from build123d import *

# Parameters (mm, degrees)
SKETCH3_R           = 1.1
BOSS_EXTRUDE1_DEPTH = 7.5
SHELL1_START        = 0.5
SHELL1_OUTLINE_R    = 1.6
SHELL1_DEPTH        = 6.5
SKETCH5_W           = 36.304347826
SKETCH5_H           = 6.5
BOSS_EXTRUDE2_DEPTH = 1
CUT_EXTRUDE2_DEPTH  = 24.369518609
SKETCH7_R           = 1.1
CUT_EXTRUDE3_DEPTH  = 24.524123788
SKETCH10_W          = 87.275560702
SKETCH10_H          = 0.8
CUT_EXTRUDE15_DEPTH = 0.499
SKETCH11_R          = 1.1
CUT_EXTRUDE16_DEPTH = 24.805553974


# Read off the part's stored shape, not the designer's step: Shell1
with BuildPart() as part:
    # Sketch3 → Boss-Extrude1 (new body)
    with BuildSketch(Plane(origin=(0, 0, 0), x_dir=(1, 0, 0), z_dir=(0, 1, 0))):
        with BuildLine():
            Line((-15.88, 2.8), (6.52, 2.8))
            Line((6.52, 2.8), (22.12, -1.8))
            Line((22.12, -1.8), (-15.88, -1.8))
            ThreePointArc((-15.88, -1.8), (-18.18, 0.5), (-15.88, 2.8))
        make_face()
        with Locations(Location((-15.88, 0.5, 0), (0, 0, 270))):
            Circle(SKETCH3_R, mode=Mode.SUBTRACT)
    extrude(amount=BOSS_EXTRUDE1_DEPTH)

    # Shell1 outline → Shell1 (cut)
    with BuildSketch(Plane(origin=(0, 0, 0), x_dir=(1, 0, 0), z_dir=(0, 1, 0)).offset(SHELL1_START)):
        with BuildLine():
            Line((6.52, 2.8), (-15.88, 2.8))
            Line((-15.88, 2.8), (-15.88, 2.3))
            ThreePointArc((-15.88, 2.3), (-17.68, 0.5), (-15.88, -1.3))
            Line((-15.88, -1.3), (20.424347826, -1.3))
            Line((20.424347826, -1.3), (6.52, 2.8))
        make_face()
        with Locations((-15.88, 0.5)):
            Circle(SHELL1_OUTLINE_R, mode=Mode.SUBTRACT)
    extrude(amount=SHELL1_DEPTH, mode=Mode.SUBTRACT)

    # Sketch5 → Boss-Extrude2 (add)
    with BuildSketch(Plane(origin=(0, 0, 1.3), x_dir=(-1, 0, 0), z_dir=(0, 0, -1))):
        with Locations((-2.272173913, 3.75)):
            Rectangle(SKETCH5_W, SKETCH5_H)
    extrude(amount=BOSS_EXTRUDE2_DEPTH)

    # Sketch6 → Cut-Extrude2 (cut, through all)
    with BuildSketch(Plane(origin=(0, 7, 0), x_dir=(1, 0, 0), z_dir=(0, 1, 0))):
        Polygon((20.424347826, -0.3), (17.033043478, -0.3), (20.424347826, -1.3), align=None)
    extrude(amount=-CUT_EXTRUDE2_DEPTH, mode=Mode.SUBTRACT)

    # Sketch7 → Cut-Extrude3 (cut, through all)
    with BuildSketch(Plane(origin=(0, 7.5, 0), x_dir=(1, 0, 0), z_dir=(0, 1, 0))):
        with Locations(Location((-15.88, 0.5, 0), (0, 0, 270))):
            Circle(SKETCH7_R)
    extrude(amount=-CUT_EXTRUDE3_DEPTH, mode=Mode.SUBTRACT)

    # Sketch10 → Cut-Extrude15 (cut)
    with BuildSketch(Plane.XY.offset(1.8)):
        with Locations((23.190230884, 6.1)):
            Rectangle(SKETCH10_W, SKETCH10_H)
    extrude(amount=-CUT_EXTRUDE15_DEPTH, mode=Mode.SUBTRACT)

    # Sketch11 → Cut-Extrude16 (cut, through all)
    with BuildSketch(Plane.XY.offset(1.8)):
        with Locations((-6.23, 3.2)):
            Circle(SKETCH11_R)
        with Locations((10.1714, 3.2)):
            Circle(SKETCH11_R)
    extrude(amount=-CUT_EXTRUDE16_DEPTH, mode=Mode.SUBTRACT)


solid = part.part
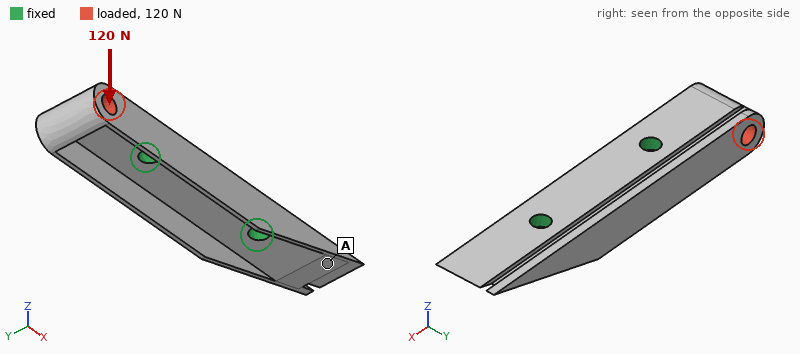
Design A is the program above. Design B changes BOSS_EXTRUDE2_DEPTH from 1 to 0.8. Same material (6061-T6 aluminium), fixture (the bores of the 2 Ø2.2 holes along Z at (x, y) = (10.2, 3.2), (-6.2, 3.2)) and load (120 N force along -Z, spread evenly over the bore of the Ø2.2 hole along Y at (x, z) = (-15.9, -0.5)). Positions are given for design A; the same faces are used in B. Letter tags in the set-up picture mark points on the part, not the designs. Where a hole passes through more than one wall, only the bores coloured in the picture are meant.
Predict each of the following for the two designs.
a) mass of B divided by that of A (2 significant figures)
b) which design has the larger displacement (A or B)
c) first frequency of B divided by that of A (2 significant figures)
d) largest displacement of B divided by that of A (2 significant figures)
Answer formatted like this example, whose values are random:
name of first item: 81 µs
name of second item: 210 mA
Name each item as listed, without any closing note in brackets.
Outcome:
mass of B divided by that of A: 0.92
which design has the larger displacement: B
first frequency of B divided by that of A: 0.93
largest displacement of B divided by that of A: 1.2
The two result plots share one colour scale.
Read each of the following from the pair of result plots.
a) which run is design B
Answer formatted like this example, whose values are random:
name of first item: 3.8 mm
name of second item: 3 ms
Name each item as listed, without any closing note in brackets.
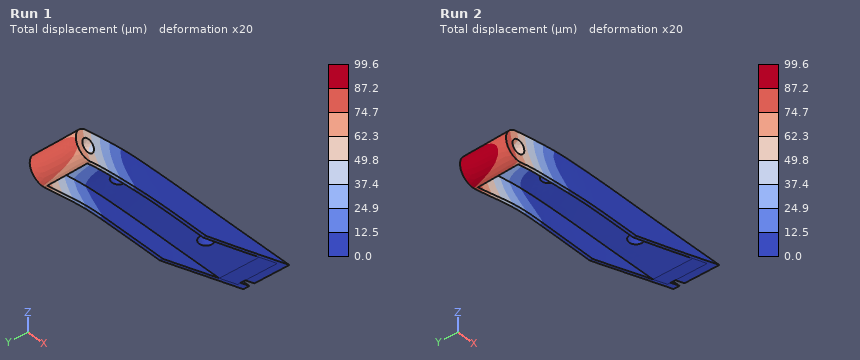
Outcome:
which run is design B: Run 2
